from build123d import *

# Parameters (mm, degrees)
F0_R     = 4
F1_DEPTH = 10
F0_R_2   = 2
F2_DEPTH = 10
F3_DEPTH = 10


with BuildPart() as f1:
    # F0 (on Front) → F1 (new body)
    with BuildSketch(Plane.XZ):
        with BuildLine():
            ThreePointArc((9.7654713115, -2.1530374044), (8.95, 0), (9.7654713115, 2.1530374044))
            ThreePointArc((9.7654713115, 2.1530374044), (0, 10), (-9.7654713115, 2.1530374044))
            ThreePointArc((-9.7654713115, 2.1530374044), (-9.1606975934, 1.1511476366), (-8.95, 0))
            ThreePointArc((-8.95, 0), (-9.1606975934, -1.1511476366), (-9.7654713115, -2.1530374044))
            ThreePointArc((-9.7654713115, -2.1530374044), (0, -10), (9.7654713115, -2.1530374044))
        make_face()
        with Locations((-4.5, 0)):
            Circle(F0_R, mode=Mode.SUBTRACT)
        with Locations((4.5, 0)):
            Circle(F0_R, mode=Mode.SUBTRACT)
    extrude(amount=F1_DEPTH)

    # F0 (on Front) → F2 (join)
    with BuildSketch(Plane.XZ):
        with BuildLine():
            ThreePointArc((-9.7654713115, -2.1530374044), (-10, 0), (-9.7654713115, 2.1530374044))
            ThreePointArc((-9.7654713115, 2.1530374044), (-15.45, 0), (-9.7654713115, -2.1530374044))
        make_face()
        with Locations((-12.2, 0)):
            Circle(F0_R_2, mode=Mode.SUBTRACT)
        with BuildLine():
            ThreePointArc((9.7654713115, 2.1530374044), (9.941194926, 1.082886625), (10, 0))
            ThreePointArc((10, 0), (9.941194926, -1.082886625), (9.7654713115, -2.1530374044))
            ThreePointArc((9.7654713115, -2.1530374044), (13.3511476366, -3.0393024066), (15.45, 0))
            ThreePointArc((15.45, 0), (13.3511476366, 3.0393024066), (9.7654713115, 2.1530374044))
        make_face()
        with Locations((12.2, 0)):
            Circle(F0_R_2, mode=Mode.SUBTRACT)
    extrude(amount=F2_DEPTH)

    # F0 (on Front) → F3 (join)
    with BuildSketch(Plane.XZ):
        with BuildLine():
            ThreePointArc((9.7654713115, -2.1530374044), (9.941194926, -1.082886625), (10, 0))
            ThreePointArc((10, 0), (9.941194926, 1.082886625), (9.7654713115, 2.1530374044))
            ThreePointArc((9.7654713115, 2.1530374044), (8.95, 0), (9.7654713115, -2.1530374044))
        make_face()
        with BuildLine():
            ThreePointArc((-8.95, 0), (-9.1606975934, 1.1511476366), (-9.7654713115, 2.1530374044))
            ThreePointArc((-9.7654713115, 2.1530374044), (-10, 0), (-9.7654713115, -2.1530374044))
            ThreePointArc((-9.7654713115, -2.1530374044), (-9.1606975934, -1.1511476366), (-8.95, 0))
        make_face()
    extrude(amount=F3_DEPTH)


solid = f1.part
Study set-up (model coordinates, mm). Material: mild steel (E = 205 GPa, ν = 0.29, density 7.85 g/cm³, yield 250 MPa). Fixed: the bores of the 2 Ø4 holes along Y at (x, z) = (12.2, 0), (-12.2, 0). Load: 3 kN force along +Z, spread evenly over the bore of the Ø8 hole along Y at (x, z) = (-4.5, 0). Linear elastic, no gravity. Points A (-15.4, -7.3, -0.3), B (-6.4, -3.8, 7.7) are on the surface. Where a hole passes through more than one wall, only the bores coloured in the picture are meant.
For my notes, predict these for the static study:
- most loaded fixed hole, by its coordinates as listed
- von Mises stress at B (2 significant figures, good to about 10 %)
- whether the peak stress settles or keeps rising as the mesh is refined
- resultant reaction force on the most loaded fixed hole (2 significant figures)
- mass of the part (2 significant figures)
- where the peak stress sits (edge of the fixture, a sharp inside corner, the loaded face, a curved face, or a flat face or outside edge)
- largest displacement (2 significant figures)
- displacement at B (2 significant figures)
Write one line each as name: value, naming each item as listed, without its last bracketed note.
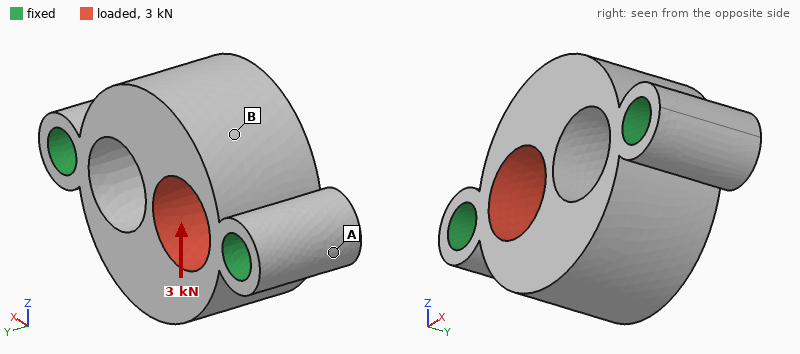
most loaded fixed hole, by its coordinates as listed: (-12.2, 0)
von Mises stress at B: 31 MPa
whether the peak stress settles or keeps rising as the mesh is refined: keeps rising
resultant reaction force on the most loaded fixed hole: 2.2 kN
mass of the part: 20 g
where the peak stress sits: edge of the fixture
largest displacement: 2.9 µm
displacement at B: 2.4 µm
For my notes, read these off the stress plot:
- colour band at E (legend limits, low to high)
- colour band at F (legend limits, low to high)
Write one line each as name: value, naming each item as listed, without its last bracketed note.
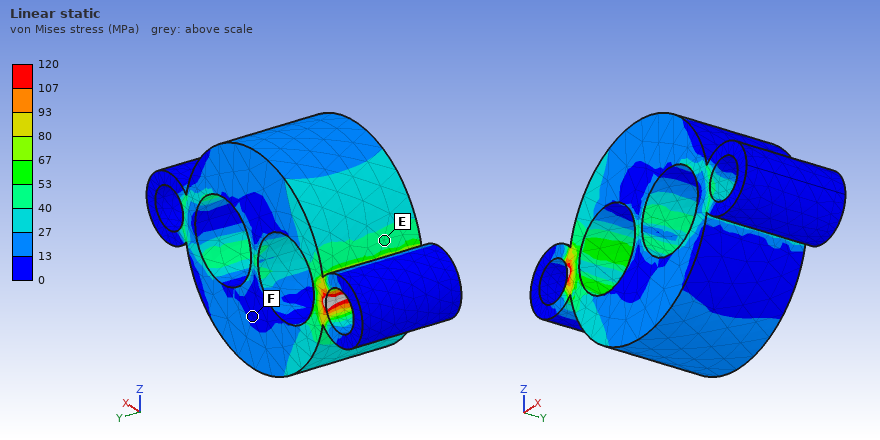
colour band at E: 40 to 53 MPa
colour band at F: 0 to 13 MPa
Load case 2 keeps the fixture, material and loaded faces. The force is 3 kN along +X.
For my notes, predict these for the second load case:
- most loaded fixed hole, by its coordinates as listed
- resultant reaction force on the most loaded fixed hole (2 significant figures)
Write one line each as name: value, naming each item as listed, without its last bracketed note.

most loaded fixed hole, by its coordinates as listed: (-12.2, 0)
resultant reaction force on the most loaded fixed hole: 2.0 kN
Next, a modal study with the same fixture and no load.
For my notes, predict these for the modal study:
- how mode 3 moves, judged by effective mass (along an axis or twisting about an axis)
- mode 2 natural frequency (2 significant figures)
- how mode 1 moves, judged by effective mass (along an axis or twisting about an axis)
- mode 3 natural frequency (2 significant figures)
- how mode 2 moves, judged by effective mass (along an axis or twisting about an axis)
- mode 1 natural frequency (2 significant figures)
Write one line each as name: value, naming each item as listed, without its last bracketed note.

how mode 3 moves, judged by effective mass: along X
mode 2 natural frequency: 31 kHz
how mode 1 moves, judged by effective mass: twisting about X
mode 3 natural frequency: 36 kHz
how mode 2 moves, judged by effective mass: along Y
mode 1 natural frequency: 27 kHz
